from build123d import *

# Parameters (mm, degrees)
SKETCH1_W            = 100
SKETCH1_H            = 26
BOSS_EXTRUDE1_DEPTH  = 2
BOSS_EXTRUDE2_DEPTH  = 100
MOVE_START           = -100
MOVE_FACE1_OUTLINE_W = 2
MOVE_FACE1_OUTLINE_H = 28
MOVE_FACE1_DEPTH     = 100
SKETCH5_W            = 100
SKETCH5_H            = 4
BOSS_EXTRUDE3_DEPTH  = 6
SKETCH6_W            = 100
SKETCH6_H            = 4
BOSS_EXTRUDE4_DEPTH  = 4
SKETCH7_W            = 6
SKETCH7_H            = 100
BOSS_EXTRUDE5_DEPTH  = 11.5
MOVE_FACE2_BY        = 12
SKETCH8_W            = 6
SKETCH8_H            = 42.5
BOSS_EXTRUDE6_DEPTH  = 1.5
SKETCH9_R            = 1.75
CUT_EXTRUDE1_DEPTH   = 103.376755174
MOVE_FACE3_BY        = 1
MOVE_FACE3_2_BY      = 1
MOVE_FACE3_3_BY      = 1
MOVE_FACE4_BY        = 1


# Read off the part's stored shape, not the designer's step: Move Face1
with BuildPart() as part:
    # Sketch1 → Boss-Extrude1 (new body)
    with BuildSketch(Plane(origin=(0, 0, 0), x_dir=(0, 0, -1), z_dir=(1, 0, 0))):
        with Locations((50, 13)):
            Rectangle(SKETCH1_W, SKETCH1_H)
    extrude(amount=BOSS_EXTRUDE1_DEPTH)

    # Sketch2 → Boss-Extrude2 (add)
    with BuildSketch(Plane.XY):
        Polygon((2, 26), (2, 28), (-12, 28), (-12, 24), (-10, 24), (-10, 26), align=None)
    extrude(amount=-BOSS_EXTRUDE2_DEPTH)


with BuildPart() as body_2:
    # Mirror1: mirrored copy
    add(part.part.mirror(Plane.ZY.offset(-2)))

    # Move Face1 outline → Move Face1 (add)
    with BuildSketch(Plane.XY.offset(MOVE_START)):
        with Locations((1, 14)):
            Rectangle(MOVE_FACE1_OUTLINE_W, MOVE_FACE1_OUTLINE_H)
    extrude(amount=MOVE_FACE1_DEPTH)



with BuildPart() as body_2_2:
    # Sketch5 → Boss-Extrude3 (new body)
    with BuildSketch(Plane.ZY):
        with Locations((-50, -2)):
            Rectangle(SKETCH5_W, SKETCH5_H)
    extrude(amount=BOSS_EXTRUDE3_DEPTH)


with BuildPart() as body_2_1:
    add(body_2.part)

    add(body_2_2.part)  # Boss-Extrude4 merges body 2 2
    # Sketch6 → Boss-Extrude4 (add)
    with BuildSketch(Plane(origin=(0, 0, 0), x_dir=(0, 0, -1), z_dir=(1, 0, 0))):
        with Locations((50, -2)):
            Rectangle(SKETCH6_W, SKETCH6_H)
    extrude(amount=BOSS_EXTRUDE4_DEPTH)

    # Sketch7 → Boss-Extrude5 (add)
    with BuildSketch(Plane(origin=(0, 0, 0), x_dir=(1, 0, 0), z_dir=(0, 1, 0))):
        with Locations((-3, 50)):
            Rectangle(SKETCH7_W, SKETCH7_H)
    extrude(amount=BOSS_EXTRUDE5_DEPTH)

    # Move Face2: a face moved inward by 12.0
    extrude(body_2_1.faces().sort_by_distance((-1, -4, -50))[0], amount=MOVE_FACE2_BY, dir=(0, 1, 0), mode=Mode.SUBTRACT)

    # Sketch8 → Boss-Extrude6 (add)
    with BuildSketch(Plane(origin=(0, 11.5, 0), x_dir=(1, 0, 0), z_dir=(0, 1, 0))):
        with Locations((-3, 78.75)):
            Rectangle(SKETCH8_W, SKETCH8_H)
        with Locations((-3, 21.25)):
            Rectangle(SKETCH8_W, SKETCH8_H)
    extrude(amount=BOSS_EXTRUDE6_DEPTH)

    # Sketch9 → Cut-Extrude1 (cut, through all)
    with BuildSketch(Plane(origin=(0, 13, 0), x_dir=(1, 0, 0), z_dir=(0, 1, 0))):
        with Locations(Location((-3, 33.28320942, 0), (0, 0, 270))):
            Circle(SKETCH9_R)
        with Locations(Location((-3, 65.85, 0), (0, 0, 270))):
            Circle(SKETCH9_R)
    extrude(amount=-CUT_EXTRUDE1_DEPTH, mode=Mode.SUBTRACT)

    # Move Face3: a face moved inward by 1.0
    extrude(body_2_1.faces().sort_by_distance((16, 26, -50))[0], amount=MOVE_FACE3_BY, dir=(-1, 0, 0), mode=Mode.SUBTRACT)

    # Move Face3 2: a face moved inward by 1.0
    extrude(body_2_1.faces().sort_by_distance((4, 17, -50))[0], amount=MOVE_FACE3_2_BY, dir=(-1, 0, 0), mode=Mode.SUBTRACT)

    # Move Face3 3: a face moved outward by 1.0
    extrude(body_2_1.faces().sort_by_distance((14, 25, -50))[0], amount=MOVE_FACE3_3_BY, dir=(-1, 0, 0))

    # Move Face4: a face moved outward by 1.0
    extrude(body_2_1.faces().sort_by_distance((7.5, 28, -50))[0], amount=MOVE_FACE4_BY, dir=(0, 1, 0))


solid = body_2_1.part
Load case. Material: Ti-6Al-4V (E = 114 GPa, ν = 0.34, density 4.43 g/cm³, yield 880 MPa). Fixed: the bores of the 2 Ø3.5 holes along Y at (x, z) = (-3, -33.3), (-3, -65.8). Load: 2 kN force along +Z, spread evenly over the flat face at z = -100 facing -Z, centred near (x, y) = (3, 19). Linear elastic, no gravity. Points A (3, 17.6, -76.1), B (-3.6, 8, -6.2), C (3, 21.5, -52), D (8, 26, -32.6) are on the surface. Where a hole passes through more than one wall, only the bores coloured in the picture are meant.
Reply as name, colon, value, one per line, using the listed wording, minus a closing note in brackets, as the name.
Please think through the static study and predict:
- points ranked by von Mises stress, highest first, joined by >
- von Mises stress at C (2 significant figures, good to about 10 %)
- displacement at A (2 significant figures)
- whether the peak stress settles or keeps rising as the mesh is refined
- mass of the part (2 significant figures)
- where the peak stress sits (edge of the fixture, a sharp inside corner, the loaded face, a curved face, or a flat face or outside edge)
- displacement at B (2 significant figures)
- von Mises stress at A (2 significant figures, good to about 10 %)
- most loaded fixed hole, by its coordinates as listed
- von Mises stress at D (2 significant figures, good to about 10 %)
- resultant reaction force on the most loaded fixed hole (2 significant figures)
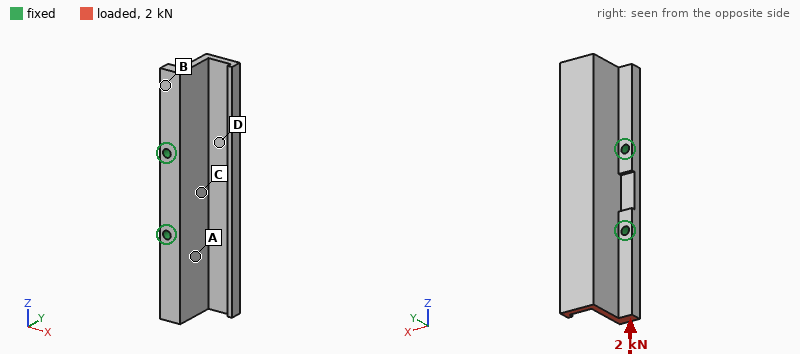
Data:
points ranked by von Mises stress, highest first, joined by >: C > A > D > B
von Mises stress at C: 28 MPa
displacement at A: 9.8 µm
whether the peak stress settles or keeps rising as the mesh is refined: keeps rising
mass of the part: 58 g
where the peak stress sits: edge of the fixture
displacement at B: 12 µm
von Mises stress at A: 18 MPa
most loaded fixed hole, by its coordinates as listed: (-3, -65.8)
von Mises stress at D: 10 MPa
resultant reaction force on the most loaded fixed hole: 1.4 kN
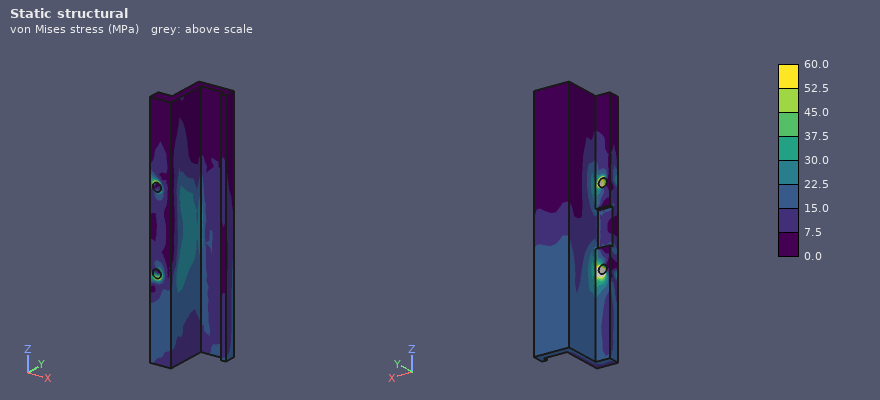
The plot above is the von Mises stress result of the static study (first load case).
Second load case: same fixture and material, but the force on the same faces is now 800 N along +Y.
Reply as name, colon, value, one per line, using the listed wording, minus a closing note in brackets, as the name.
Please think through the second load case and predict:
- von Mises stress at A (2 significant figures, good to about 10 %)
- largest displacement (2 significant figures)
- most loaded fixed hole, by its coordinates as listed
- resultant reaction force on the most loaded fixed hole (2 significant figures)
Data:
von Mises stress at A: 43 MPa
largest displacement: 0.19 mm
most loaded fixed hole, by its coordinates as listed: (-3, -65.8)
resultant reaction force on the most loaded fixed hole: 1.6 kN
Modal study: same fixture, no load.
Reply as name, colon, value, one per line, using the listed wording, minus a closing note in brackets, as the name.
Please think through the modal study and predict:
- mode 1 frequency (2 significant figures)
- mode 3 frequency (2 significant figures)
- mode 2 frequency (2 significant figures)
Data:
mode 1 frequency: 2500 Hz
mode 3 frequency: 5300 Hz
mode 2 frequency: 2600 Hz
